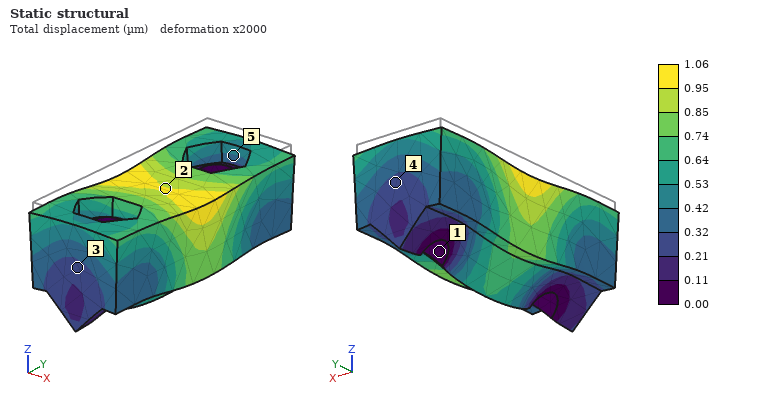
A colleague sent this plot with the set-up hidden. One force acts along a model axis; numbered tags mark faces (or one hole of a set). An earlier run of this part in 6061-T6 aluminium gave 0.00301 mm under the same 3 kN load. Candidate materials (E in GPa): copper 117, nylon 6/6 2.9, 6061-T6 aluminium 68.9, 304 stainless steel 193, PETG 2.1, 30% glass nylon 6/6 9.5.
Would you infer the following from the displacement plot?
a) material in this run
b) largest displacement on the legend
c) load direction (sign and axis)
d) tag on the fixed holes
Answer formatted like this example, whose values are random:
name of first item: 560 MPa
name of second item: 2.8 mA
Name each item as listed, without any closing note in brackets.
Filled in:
material in this run: 304 stainless steel
largest displacement on the legend: 1.06 µm
load direction: -Z
tag on the fixed holes: 1
